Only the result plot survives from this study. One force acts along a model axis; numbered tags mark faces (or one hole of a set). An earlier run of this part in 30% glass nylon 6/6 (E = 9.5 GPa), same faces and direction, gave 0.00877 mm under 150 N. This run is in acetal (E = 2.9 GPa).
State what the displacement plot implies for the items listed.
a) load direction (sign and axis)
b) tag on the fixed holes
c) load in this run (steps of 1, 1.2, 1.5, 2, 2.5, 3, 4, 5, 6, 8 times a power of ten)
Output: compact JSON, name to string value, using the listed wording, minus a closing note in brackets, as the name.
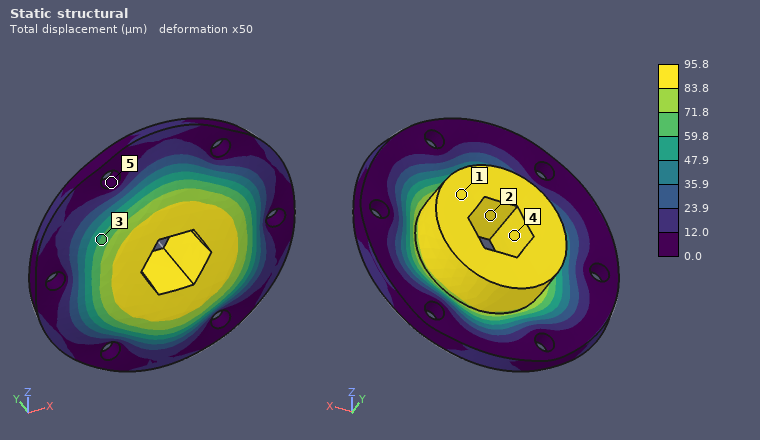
{"load direction": "-Y", "tag on the fixed holes": "5", "load in this run": "500 N"}
